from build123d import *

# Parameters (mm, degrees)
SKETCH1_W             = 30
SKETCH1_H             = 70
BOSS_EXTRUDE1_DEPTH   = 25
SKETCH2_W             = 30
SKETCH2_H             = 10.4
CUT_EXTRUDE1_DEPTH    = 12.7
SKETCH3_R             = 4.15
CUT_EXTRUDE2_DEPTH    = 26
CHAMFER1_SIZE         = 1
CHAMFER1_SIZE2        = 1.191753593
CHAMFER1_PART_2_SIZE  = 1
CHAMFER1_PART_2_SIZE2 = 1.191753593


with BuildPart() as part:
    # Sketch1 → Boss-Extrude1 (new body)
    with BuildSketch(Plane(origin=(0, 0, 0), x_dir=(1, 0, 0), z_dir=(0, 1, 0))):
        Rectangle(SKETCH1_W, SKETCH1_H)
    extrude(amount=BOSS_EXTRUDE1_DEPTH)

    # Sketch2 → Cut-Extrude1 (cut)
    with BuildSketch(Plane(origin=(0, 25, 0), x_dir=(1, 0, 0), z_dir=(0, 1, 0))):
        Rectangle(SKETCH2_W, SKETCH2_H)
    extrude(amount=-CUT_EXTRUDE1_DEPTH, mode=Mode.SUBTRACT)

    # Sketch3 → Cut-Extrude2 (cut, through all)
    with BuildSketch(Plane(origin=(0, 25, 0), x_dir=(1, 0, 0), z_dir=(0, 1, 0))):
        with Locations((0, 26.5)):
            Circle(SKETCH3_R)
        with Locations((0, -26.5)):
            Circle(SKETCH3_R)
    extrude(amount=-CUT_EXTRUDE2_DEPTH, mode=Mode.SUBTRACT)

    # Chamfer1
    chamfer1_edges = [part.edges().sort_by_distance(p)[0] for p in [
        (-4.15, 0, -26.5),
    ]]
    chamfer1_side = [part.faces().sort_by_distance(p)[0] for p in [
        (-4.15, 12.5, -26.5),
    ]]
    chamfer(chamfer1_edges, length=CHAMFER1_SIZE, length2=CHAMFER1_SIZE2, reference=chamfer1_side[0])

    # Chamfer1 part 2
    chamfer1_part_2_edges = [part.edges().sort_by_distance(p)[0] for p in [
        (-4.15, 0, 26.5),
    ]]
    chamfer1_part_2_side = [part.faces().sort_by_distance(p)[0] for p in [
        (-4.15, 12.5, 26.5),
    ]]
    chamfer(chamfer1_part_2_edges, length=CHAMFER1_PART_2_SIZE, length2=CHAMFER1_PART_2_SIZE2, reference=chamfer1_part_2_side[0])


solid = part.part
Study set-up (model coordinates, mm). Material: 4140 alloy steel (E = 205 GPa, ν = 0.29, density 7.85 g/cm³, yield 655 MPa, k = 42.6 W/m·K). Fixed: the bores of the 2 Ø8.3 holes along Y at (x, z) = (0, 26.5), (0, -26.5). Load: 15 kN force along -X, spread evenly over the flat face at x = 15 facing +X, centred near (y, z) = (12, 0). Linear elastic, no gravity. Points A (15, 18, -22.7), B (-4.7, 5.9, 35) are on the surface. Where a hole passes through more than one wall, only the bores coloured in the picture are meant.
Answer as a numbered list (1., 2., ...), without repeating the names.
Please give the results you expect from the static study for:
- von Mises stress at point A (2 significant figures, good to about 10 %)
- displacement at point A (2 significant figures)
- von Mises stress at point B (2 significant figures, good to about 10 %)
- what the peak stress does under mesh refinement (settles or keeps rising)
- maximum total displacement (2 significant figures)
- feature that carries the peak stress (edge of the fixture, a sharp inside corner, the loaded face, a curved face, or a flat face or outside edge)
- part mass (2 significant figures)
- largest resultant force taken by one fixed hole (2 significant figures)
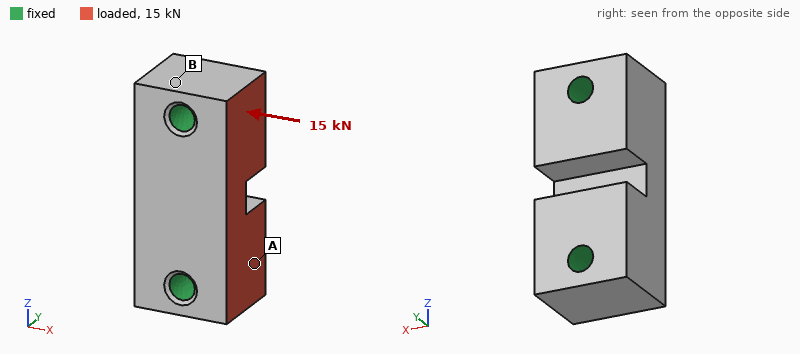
1. 13 MPa
2. 1.4 µm
3. 6.0 MPa
4. keeps rising
5. 3.1 µm
6. edge of the fixture
7. 360 g
8. 7.5 kN
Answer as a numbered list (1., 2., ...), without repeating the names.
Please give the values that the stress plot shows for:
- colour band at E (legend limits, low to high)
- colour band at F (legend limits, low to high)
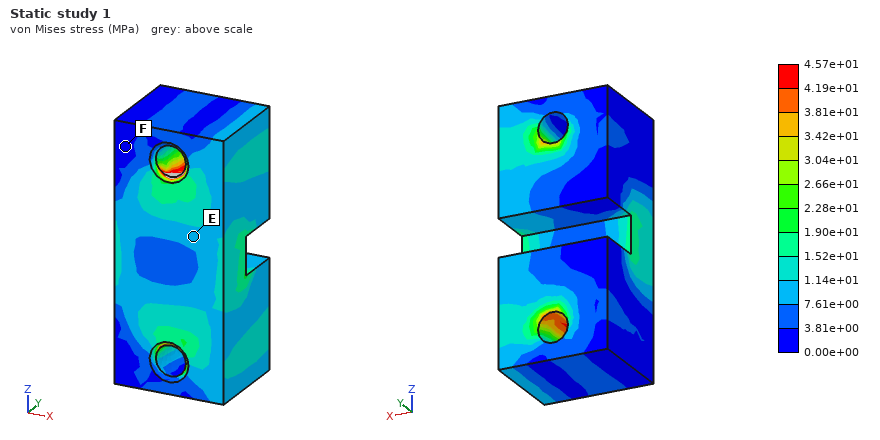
1. 7.61e+00 to 1.14e+01 MPa
2. 0.00e+00 to 3.81e+00 MPa
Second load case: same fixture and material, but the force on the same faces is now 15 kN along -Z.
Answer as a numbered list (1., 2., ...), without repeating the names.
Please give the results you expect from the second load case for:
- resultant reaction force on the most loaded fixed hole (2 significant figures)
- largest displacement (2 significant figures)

1. 8.1 kN
2. 4.2 µm
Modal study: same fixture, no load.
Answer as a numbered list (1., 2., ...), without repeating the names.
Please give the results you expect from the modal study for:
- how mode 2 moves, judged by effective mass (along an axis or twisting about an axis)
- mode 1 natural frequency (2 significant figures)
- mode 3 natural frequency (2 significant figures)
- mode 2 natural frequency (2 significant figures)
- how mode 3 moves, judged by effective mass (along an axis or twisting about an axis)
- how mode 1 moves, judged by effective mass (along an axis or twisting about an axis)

1. along Y
2. 21 kHz
3. 29 kHz
4. 24 kHz
5. twisting about Z
6. along X
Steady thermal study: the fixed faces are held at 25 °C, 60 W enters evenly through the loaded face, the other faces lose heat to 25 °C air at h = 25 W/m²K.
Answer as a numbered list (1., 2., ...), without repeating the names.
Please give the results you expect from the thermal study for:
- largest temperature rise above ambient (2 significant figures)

1. 19 K
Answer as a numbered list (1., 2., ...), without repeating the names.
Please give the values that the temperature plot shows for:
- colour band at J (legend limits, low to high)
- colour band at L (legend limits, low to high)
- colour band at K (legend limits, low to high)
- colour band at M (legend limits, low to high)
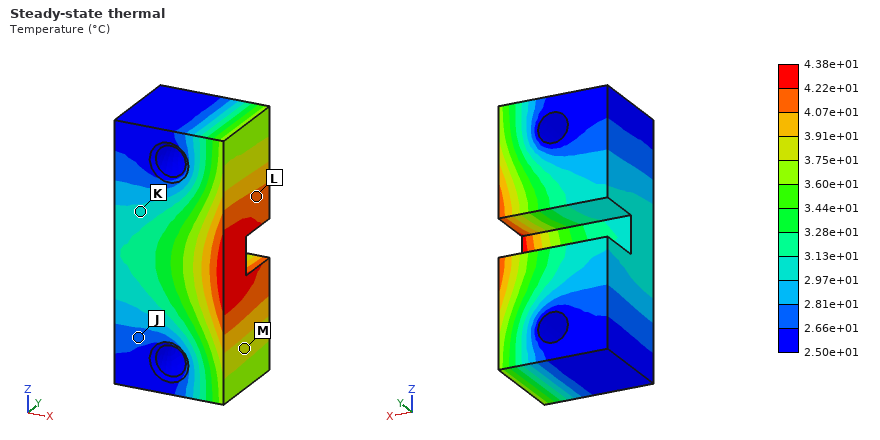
1. 2.66e+01 to 2.81e+01 °C
2. 4.07e+01 to 4.22e+01 °C
3. 2.97e+01 to 3.13e+01 °C
4. 3.75e+01 to 3.91e+01 °C
